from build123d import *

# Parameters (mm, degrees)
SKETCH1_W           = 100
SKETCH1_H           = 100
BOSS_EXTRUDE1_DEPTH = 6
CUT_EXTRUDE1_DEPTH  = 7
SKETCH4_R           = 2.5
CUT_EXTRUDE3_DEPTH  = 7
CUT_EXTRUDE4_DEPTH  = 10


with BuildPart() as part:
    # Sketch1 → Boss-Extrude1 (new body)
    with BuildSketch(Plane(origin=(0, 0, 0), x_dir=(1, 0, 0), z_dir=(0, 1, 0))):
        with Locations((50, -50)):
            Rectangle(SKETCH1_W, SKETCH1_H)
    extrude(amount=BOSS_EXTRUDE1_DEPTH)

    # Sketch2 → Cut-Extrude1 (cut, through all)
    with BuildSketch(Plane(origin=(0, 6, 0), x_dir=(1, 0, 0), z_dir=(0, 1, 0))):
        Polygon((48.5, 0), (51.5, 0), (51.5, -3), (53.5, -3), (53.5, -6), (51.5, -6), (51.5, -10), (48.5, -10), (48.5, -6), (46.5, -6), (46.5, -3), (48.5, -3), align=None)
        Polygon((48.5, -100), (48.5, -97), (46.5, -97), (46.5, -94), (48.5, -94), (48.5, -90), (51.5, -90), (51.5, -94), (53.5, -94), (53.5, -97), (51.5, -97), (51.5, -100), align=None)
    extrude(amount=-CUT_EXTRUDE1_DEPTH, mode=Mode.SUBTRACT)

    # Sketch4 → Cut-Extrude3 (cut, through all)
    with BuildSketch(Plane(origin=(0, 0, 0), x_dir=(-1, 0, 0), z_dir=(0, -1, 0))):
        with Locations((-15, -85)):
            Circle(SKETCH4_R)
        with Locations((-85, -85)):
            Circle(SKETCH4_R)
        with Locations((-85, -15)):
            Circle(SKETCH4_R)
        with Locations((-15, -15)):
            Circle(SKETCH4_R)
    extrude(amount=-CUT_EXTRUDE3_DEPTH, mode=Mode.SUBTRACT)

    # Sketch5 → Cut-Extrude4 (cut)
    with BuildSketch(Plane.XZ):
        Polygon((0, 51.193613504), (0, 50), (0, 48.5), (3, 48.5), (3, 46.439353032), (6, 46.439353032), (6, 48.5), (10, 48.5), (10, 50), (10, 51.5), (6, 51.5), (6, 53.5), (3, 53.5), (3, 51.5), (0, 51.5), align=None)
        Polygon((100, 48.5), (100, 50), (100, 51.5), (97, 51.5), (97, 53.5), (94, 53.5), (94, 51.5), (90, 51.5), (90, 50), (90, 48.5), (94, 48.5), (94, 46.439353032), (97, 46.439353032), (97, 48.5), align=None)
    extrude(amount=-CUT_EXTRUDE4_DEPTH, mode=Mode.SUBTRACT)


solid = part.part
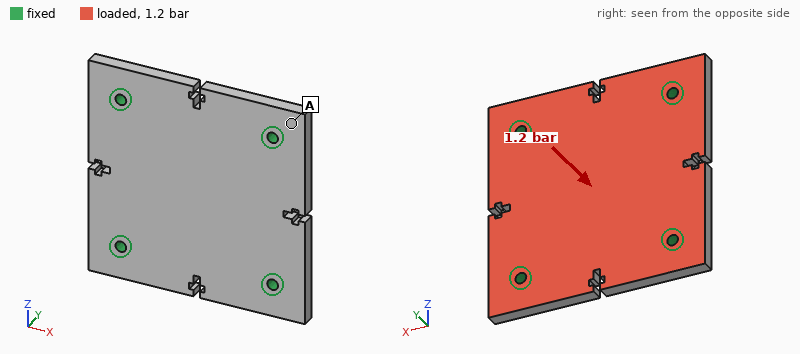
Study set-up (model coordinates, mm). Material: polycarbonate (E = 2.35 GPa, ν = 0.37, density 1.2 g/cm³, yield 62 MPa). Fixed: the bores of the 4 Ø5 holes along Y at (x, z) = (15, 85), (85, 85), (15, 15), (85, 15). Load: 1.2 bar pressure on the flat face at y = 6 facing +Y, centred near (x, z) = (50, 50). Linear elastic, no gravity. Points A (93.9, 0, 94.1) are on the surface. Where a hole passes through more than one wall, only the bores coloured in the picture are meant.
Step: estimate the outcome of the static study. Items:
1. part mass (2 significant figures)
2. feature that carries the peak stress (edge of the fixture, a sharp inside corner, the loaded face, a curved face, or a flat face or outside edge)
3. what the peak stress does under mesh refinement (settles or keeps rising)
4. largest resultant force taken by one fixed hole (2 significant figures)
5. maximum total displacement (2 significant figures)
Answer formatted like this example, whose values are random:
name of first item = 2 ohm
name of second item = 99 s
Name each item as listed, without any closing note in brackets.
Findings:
part mass = 70 g
feature that carries the peak stress = edge of the fixture
what the peak stress does under mesh refinement = keeps rising
largest resultant force taken by one fixed hole = 290 N
maximum total displacement = 0.44 mm
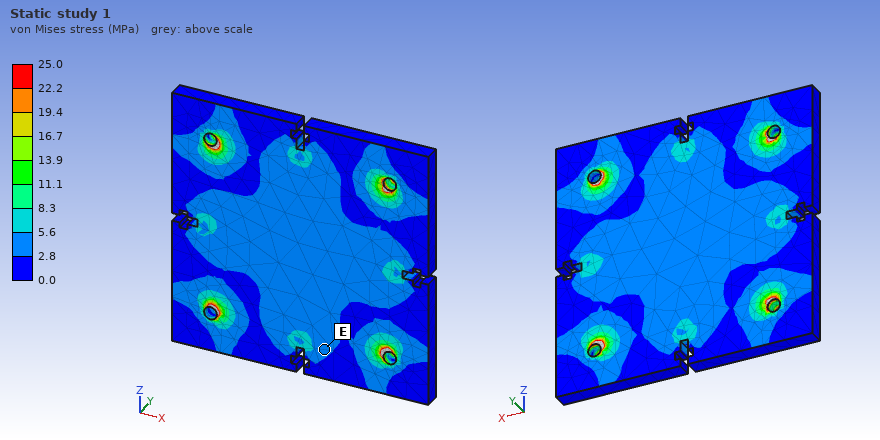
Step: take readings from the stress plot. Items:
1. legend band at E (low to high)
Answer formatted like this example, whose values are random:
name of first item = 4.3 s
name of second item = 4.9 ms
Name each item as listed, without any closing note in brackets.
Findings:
legend band at E = 2.8 to 5.6 MPa
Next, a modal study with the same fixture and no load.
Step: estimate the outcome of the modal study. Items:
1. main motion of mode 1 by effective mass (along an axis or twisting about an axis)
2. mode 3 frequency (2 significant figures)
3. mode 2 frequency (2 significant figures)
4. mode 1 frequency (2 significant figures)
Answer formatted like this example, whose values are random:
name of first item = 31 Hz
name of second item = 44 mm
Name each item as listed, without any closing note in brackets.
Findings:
main motion of mode 1 by effective mass = along Y
mode 3 frequency = 1700 Hz
mode 2 frequency = 1600 Hz
mode 1 frequency = 1200 Hz
